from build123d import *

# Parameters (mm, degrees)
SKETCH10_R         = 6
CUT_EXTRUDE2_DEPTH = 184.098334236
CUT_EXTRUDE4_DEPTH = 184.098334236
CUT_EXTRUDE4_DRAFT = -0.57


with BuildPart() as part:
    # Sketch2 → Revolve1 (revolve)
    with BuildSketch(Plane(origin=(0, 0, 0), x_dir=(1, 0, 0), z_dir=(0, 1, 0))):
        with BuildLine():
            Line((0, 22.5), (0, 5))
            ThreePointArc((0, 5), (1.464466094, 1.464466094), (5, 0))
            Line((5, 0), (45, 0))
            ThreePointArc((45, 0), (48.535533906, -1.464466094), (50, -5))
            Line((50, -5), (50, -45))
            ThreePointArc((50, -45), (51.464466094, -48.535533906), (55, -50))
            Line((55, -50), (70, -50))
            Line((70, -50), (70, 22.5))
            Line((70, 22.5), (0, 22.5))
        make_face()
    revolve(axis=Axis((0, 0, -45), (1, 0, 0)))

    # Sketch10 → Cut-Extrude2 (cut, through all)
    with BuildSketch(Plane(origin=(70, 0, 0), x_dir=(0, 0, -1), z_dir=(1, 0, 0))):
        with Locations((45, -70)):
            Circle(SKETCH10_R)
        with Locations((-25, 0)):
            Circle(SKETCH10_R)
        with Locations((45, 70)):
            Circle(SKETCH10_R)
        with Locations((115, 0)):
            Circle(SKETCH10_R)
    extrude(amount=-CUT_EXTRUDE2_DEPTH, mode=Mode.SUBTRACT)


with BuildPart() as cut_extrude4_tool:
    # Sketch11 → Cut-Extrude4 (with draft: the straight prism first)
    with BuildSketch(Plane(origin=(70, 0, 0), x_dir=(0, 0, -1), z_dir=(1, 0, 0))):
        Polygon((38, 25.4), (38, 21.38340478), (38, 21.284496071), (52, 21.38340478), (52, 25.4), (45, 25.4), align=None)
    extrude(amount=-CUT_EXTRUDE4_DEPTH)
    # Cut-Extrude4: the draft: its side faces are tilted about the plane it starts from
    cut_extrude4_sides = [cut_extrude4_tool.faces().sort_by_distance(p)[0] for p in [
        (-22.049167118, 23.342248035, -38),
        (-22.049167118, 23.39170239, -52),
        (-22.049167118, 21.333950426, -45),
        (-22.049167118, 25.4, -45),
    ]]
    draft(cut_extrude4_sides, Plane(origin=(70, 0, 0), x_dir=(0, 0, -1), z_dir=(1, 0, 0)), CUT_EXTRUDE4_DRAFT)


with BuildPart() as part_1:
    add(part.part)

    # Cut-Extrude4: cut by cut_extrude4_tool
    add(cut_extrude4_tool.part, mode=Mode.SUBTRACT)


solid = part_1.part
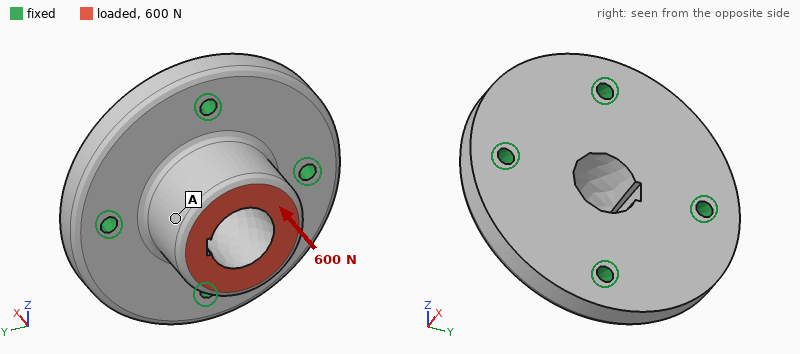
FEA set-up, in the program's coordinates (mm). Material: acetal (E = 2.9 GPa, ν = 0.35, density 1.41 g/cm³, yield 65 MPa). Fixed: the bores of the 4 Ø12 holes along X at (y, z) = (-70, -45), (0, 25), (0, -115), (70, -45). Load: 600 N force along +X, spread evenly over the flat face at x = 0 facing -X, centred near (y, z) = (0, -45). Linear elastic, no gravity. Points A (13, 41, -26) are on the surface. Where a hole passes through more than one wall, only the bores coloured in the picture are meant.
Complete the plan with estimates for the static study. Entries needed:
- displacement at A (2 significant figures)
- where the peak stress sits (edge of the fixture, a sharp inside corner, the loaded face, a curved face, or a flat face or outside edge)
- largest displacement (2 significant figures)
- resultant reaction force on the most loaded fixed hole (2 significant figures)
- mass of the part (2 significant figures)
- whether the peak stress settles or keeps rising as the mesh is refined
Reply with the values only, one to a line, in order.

10 µm
edge of the fixture
11 µm
160 N
1.1 kg
keeps rising
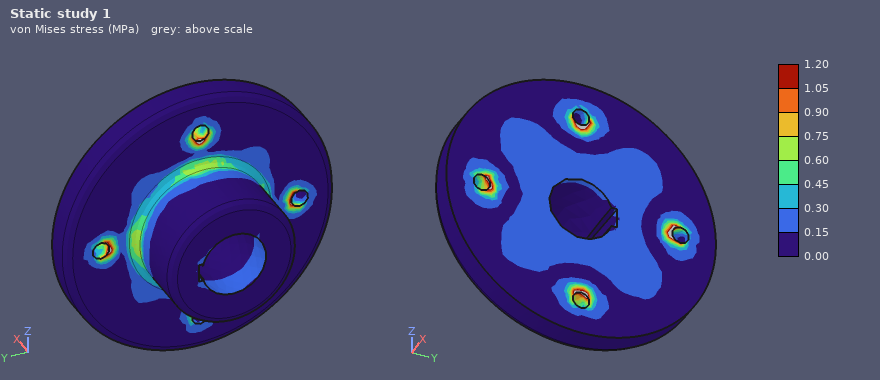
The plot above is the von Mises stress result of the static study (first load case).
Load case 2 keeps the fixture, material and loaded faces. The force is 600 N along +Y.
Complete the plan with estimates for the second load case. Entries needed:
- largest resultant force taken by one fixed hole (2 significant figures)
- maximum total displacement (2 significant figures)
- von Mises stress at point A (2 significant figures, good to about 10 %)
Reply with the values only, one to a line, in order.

340 N
35 µm
0.26 MPa
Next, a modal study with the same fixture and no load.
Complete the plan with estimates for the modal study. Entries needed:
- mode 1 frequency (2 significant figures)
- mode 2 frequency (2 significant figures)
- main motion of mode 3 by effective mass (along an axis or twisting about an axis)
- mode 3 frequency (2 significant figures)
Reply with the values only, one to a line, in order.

1500 Hz
1500 Hz
along X
1600 Hz
